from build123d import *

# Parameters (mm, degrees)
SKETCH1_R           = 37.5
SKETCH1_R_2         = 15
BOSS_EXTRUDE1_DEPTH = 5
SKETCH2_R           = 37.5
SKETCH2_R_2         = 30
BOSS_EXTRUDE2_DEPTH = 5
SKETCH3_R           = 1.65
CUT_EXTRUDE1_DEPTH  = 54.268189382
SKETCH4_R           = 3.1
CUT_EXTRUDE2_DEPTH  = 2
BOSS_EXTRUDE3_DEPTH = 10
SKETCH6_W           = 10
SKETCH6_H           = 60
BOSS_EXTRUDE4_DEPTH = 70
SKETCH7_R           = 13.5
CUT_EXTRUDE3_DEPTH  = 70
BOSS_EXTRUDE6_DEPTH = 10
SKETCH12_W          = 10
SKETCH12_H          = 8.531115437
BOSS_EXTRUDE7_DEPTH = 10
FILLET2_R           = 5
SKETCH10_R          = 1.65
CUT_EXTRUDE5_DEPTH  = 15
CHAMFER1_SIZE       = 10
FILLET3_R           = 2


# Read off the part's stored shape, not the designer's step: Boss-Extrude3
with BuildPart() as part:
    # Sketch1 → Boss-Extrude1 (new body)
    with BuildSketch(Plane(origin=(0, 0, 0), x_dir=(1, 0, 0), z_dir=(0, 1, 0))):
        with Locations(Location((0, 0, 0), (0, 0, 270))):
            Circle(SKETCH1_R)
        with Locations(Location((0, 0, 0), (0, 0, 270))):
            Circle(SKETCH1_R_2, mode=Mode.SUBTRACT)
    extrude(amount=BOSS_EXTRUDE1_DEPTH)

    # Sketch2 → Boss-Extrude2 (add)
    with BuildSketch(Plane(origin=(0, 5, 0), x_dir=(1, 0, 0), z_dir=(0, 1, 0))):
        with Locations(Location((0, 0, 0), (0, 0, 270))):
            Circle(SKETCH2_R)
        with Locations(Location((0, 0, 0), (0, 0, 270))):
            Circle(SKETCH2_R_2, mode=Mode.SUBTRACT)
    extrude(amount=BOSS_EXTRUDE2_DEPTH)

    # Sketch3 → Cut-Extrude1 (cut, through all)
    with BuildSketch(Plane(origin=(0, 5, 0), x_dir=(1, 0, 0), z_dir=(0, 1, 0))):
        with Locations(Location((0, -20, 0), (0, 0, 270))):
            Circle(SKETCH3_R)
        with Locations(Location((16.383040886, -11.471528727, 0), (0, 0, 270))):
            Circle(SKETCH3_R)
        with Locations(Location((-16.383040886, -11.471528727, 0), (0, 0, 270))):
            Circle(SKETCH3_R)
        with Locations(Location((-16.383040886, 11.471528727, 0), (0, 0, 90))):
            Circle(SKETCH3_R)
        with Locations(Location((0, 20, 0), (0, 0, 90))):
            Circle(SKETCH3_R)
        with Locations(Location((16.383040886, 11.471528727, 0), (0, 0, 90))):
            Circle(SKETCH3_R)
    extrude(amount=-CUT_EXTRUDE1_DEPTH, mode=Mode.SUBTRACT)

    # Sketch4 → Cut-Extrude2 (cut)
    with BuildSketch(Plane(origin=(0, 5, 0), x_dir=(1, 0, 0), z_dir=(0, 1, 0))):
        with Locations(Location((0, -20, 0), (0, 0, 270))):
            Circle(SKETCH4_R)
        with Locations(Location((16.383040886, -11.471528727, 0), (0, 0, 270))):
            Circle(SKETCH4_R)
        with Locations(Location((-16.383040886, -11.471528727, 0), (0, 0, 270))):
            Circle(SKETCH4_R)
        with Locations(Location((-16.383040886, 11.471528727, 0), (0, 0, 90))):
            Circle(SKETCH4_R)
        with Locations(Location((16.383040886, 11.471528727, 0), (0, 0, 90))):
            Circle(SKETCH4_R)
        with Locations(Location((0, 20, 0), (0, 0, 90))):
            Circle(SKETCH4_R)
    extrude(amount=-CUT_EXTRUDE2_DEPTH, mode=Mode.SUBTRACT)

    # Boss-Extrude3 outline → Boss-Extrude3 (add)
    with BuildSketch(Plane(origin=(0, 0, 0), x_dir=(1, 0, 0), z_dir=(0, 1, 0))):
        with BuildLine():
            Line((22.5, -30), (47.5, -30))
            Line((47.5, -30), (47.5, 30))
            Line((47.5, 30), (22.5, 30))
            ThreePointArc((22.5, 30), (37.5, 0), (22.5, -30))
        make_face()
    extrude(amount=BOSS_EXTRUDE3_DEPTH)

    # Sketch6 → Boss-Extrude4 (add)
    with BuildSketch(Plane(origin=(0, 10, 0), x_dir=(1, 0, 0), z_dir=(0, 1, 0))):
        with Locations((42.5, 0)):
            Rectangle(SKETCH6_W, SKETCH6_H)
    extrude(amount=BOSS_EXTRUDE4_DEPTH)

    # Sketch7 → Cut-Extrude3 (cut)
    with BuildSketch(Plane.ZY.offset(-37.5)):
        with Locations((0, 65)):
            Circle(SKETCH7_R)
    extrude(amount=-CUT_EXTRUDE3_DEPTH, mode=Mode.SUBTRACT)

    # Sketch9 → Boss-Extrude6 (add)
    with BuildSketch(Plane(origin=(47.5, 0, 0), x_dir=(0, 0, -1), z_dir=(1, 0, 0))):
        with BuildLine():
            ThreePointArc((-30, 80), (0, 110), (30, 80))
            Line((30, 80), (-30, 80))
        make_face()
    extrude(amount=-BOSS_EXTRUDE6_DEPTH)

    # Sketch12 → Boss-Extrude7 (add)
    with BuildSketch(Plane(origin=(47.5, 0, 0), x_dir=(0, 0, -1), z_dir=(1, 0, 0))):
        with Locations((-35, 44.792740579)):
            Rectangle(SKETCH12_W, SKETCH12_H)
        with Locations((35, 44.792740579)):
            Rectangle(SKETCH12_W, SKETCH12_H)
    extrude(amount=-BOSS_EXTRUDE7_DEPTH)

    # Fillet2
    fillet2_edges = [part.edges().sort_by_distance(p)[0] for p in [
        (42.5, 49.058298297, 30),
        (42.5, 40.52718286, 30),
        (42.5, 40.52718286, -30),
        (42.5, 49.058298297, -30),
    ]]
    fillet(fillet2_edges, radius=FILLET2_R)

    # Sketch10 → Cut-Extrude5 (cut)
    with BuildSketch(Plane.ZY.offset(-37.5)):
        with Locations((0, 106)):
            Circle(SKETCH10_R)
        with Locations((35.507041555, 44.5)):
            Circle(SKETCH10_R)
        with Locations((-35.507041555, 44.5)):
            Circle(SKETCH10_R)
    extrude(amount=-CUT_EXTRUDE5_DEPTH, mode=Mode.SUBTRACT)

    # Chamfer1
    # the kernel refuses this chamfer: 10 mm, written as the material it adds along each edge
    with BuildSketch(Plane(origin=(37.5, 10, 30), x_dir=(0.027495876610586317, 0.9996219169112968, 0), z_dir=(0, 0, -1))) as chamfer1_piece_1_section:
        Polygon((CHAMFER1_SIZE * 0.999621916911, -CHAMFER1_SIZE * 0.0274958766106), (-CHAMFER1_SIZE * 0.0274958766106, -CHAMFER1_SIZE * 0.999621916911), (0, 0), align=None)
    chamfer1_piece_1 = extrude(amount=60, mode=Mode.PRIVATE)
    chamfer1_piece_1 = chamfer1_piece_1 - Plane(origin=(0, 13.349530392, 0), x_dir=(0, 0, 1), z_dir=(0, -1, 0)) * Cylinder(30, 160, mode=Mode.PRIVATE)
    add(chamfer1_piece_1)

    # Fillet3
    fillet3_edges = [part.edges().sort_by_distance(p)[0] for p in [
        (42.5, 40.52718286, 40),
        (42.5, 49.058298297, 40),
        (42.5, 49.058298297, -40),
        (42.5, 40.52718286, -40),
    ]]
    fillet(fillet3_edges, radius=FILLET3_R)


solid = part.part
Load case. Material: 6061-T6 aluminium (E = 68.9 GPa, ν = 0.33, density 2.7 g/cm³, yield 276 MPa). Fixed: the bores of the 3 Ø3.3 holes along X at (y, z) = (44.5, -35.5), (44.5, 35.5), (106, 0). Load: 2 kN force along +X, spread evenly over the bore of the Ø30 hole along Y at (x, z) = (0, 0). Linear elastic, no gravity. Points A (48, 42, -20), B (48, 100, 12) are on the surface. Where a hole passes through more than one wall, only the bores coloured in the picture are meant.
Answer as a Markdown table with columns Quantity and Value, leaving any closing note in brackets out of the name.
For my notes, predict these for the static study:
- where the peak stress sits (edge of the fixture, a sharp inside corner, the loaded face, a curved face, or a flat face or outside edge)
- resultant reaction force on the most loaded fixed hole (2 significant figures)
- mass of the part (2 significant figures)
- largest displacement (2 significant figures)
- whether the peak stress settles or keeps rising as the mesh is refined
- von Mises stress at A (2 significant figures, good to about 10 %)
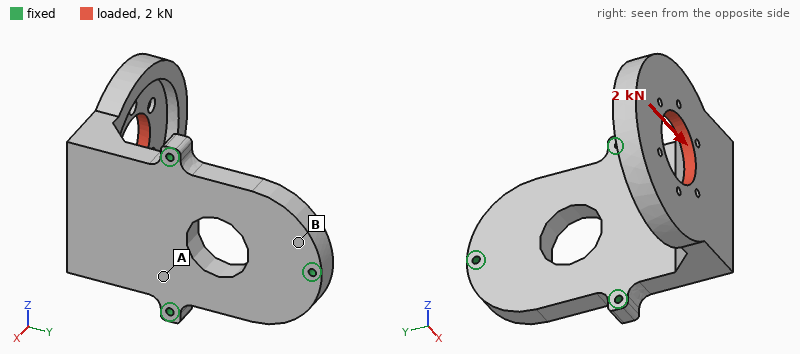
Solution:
| Quantity | Value |
|---|---|
| where the peak stress sits | edge of the fixture |
| resultant reaction force on the most loaded fixed hole | 1.4 kN |
| mass of the part | 240 g |
| largest displacement | 0.78 mm |
| whether the peak stress settles or keeps rising as the mesh is refined | keeps rising |
| von Mises stress at A | 68 MPa |
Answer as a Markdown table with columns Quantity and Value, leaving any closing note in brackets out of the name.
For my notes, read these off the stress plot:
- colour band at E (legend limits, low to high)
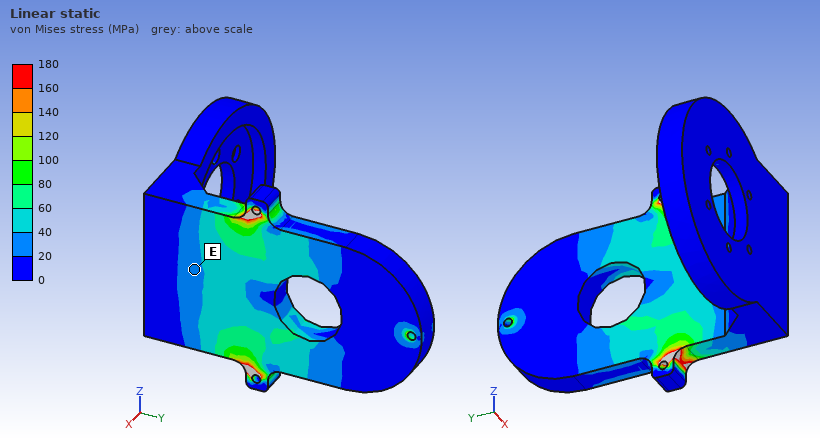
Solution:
| Quantity | Value |
|---|---|
| colour band at E | 20 to 40 MPa |
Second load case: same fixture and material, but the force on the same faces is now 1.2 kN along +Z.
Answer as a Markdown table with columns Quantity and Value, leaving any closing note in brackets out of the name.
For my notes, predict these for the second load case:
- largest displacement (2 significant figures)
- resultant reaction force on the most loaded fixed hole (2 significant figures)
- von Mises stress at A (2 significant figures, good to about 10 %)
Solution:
| Quantity | Value |
|---|---|
| largest displacement | 0.19 mm |
| resultant reaction force on the most loaded fixed hole | 1.3 kN |
| von Mises stress at A | 21 MPa |
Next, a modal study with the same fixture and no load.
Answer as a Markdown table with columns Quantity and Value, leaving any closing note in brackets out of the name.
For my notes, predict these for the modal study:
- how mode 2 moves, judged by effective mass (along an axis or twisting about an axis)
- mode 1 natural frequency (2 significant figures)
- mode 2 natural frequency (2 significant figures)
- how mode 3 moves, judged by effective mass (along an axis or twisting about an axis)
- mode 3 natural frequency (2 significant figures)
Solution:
| Quantity | Value |
|---|---|
| how mode 2 moves, judged by effective mass | along Z |
| mode 1 natural frequency | 760 Hz |
| mode 2 natural frequency | 1600 Hz |
| how mode 3 moves, judged by effective mass | along X |
| mode 3 natural frequency | 1900 Hz |
